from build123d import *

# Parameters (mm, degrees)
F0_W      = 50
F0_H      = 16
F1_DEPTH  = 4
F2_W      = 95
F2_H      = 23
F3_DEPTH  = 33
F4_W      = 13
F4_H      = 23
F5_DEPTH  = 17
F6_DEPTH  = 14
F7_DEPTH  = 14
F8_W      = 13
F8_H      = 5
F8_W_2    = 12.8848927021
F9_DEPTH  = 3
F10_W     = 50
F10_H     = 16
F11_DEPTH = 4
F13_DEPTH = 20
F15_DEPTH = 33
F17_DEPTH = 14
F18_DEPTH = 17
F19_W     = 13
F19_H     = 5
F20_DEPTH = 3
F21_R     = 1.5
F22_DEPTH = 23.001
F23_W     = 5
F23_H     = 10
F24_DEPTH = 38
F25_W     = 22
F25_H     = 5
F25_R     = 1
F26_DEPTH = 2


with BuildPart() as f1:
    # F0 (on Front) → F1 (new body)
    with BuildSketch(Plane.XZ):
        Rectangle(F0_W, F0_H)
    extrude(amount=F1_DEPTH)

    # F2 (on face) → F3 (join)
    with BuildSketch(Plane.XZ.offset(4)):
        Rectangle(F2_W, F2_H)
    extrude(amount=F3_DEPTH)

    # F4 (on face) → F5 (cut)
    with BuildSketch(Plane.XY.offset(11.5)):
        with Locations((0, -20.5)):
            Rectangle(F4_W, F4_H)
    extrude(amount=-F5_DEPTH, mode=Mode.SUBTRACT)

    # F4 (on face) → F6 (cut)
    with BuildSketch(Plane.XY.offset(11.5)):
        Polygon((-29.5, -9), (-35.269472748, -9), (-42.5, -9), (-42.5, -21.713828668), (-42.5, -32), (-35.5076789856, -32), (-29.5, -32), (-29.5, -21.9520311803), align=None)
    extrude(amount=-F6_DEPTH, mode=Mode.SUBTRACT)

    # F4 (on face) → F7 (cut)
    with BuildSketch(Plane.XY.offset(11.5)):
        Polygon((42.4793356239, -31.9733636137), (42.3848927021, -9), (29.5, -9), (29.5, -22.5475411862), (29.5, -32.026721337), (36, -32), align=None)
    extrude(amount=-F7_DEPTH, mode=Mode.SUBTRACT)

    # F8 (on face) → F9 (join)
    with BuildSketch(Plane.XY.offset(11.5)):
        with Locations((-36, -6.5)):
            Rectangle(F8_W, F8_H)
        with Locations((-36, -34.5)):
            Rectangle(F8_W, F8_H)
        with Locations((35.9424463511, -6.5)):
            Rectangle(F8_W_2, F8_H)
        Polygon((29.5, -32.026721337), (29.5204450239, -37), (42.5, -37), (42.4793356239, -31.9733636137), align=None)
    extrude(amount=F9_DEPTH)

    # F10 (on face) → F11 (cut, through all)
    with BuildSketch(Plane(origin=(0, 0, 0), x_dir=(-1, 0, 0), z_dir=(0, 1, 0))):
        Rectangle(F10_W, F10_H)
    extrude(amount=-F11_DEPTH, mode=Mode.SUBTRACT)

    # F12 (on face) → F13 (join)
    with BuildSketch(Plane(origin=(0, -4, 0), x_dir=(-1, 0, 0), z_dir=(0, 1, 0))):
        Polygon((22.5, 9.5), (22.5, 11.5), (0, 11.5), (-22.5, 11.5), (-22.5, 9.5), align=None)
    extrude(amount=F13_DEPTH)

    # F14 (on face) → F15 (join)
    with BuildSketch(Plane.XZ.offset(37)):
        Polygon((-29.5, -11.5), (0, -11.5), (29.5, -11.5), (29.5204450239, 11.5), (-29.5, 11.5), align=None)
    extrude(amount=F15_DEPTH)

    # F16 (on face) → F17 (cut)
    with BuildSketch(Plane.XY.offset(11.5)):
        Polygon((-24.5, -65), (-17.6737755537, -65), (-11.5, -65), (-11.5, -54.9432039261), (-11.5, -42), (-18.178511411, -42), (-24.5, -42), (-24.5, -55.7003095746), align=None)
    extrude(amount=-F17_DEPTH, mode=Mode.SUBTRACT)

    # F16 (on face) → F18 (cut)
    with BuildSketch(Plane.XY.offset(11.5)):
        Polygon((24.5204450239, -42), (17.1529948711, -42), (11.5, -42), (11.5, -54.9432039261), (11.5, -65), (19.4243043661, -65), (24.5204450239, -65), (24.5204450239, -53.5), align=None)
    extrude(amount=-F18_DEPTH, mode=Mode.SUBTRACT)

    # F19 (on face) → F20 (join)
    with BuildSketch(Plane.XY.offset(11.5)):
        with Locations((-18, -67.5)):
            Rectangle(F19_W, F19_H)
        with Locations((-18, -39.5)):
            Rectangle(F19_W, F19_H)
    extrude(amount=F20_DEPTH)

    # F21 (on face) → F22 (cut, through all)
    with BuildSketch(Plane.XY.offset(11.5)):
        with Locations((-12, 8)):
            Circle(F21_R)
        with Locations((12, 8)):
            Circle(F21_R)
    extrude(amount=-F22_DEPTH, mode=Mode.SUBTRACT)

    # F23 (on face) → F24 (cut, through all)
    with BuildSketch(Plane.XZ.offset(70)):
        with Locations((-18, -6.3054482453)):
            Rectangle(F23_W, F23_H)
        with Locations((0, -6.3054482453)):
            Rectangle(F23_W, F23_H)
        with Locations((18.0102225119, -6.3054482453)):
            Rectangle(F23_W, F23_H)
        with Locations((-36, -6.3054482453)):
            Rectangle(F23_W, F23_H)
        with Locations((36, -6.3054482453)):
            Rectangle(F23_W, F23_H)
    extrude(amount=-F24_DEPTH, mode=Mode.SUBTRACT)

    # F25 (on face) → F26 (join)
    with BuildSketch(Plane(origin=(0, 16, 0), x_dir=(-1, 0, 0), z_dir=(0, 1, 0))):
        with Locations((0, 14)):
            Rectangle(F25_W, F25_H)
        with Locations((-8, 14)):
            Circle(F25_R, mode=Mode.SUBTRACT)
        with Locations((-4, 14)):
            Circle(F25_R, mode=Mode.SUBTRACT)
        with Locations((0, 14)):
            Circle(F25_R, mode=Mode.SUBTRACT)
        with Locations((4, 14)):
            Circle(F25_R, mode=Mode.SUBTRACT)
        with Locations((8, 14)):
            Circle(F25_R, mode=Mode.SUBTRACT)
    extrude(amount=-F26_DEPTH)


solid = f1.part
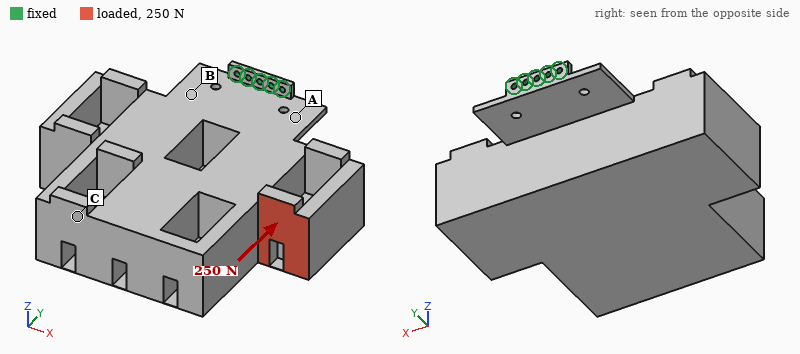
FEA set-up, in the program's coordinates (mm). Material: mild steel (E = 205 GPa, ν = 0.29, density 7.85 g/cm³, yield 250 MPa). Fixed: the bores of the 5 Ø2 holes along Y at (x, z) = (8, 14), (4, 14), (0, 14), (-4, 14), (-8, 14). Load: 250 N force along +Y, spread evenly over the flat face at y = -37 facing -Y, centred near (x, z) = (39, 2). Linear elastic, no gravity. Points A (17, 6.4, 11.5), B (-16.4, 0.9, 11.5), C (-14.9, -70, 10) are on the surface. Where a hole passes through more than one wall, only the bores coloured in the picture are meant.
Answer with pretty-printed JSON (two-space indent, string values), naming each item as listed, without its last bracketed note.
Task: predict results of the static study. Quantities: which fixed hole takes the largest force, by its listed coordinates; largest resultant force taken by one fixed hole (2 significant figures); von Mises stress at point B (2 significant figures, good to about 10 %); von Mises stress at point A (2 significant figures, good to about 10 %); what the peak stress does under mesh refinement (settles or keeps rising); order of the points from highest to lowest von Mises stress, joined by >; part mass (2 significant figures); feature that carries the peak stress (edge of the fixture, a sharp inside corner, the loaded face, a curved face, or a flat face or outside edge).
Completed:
{
  "which fixed hole takes the largest force, by its listed coordinates": "(8, 14)",
  "largest resultant force taken by one fixed hole": "500 N",
  "von Mises stress at point B": "78 MPa",
  "von Mises stress at point A": "39 MPa",
  "what the peak stress does under mesh refinement": "keeps rising",
  "order of the points from highest to lowest von Mises stress, joined by >": "B > A > C",
  "part mass": "720 g",
  "feature that carries the peak stress": "edge of the fixture"
}
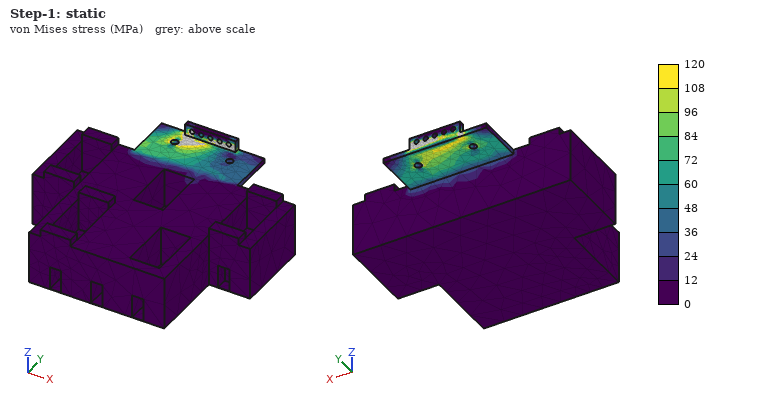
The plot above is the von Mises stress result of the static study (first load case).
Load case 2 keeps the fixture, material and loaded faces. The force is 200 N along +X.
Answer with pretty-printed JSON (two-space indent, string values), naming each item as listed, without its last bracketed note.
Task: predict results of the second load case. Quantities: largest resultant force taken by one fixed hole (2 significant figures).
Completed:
{
  "largest resultant force taken by one fixed hole": "520 N"
}
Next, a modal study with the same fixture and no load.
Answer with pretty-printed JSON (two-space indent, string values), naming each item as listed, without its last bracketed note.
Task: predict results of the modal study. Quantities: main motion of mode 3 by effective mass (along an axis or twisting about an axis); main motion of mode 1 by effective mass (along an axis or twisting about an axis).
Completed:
{
  "main motion of mode 3 by effective mass": "along X",
  "main motion of mode 1 by effective mass": "along Z"
}
